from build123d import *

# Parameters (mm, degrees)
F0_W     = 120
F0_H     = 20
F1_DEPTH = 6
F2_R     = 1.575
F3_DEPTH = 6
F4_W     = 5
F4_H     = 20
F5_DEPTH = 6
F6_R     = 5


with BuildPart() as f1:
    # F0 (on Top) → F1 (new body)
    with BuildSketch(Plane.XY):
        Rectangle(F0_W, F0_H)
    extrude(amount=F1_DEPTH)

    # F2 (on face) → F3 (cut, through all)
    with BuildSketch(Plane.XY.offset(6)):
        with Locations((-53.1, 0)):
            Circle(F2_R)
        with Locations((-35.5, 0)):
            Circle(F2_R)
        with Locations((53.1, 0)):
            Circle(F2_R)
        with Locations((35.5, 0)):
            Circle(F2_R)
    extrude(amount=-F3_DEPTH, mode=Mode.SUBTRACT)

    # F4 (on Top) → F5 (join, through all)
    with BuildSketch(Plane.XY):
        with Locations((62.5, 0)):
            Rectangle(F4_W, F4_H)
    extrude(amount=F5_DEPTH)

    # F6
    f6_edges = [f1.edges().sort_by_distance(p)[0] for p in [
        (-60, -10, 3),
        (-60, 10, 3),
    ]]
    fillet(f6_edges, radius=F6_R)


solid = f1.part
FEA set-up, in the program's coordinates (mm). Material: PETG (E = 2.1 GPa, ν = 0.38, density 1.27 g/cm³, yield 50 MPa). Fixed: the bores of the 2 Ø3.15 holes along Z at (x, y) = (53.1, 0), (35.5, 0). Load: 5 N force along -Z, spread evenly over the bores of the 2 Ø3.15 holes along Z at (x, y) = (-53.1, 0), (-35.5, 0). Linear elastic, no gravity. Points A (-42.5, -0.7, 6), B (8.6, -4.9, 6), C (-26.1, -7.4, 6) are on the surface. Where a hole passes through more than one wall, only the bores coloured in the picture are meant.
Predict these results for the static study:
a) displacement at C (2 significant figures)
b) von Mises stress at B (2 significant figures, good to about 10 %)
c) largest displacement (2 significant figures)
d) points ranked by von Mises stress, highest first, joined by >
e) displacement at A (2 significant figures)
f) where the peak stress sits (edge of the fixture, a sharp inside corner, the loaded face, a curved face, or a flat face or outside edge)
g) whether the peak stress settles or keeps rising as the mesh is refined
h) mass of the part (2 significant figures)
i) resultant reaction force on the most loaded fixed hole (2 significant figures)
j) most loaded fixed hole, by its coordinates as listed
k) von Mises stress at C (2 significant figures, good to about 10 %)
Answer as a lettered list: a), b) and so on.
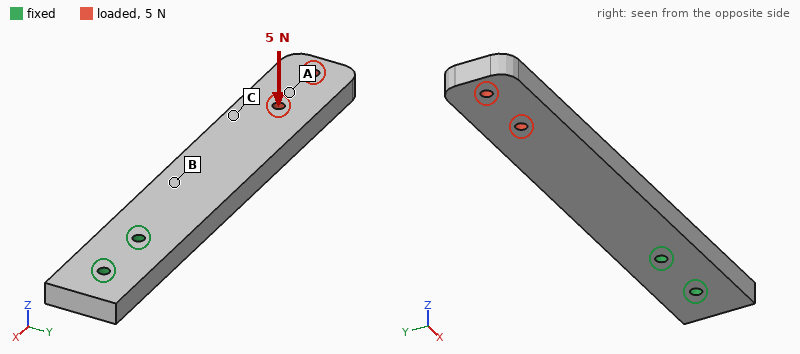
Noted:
a) 0.77 mm
b) 2.2 MPa
c) 1.5 mm
d) B > C > A
e) 1.1 mm
f) edge of the fixture
g) keeps rising
h) 19 g
i) 14 N
j) (35.5, 0)
k) 0.77 MPa
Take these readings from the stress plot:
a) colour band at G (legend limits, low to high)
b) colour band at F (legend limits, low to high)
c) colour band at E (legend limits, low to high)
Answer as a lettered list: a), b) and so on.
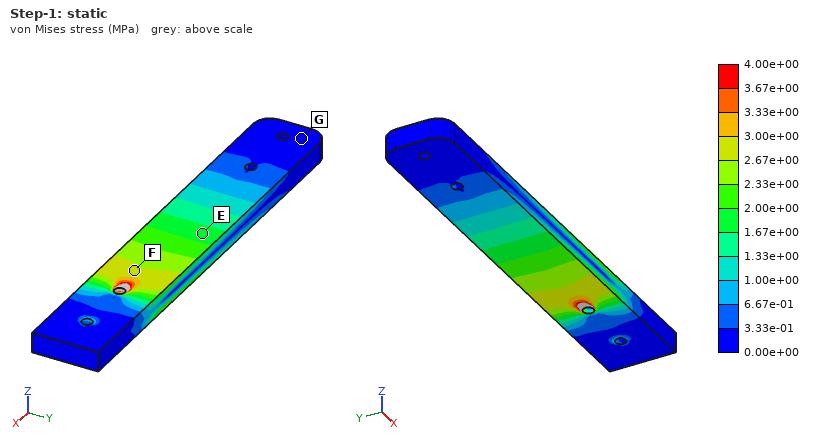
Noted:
a) 0.00e+00 to 3.33e-01 MPa
b) 2.67e+00 to 3.00e+00 MPa
c) 1.67e+00 to 2.00e+00 MPa
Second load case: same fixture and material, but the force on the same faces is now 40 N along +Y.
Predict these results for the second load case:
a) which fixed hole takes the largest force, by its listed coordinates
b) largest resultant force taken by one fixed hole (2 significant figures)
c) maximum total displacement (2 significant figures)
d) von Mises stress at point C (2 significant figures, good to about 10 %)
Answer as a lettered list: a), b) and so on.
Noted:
a) (35.5, 0)
b) 180 N
c) 1.5 mm
d) 1.4 MPa
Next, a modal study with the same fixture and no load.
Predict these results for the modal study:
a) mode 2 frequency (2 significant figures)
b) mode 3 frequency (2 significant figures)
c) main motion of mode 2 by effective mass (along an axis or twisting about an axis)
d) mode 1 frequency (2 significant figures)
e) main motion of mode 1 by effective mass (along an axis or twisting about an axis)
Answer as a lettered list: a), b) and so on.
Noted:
a) 380 Hz
b) 840 Hz
c) along Y
d) 140 Hz
e) along Z
